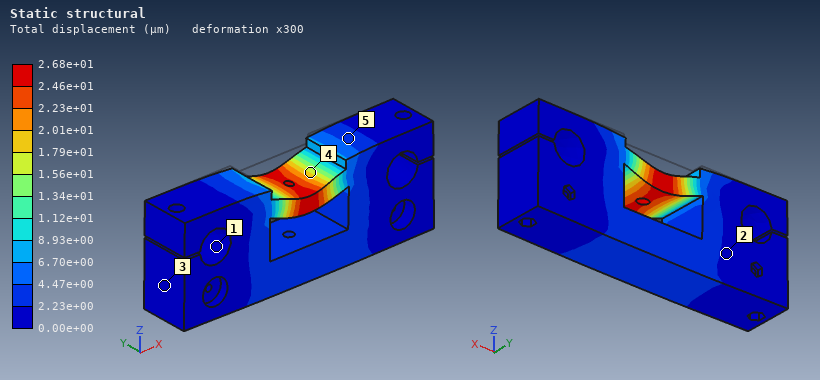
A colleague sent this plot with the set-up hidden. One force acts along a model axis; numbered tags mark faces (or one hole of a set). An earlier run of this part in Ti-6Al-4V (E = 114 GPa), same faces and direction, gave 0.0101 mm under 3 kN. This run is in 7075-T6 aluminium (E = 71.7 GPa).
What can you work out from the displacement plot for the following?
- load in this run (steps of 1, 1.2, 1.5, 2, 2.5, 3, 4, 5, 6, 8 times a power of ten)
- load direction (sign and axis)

5 kN
-Z
